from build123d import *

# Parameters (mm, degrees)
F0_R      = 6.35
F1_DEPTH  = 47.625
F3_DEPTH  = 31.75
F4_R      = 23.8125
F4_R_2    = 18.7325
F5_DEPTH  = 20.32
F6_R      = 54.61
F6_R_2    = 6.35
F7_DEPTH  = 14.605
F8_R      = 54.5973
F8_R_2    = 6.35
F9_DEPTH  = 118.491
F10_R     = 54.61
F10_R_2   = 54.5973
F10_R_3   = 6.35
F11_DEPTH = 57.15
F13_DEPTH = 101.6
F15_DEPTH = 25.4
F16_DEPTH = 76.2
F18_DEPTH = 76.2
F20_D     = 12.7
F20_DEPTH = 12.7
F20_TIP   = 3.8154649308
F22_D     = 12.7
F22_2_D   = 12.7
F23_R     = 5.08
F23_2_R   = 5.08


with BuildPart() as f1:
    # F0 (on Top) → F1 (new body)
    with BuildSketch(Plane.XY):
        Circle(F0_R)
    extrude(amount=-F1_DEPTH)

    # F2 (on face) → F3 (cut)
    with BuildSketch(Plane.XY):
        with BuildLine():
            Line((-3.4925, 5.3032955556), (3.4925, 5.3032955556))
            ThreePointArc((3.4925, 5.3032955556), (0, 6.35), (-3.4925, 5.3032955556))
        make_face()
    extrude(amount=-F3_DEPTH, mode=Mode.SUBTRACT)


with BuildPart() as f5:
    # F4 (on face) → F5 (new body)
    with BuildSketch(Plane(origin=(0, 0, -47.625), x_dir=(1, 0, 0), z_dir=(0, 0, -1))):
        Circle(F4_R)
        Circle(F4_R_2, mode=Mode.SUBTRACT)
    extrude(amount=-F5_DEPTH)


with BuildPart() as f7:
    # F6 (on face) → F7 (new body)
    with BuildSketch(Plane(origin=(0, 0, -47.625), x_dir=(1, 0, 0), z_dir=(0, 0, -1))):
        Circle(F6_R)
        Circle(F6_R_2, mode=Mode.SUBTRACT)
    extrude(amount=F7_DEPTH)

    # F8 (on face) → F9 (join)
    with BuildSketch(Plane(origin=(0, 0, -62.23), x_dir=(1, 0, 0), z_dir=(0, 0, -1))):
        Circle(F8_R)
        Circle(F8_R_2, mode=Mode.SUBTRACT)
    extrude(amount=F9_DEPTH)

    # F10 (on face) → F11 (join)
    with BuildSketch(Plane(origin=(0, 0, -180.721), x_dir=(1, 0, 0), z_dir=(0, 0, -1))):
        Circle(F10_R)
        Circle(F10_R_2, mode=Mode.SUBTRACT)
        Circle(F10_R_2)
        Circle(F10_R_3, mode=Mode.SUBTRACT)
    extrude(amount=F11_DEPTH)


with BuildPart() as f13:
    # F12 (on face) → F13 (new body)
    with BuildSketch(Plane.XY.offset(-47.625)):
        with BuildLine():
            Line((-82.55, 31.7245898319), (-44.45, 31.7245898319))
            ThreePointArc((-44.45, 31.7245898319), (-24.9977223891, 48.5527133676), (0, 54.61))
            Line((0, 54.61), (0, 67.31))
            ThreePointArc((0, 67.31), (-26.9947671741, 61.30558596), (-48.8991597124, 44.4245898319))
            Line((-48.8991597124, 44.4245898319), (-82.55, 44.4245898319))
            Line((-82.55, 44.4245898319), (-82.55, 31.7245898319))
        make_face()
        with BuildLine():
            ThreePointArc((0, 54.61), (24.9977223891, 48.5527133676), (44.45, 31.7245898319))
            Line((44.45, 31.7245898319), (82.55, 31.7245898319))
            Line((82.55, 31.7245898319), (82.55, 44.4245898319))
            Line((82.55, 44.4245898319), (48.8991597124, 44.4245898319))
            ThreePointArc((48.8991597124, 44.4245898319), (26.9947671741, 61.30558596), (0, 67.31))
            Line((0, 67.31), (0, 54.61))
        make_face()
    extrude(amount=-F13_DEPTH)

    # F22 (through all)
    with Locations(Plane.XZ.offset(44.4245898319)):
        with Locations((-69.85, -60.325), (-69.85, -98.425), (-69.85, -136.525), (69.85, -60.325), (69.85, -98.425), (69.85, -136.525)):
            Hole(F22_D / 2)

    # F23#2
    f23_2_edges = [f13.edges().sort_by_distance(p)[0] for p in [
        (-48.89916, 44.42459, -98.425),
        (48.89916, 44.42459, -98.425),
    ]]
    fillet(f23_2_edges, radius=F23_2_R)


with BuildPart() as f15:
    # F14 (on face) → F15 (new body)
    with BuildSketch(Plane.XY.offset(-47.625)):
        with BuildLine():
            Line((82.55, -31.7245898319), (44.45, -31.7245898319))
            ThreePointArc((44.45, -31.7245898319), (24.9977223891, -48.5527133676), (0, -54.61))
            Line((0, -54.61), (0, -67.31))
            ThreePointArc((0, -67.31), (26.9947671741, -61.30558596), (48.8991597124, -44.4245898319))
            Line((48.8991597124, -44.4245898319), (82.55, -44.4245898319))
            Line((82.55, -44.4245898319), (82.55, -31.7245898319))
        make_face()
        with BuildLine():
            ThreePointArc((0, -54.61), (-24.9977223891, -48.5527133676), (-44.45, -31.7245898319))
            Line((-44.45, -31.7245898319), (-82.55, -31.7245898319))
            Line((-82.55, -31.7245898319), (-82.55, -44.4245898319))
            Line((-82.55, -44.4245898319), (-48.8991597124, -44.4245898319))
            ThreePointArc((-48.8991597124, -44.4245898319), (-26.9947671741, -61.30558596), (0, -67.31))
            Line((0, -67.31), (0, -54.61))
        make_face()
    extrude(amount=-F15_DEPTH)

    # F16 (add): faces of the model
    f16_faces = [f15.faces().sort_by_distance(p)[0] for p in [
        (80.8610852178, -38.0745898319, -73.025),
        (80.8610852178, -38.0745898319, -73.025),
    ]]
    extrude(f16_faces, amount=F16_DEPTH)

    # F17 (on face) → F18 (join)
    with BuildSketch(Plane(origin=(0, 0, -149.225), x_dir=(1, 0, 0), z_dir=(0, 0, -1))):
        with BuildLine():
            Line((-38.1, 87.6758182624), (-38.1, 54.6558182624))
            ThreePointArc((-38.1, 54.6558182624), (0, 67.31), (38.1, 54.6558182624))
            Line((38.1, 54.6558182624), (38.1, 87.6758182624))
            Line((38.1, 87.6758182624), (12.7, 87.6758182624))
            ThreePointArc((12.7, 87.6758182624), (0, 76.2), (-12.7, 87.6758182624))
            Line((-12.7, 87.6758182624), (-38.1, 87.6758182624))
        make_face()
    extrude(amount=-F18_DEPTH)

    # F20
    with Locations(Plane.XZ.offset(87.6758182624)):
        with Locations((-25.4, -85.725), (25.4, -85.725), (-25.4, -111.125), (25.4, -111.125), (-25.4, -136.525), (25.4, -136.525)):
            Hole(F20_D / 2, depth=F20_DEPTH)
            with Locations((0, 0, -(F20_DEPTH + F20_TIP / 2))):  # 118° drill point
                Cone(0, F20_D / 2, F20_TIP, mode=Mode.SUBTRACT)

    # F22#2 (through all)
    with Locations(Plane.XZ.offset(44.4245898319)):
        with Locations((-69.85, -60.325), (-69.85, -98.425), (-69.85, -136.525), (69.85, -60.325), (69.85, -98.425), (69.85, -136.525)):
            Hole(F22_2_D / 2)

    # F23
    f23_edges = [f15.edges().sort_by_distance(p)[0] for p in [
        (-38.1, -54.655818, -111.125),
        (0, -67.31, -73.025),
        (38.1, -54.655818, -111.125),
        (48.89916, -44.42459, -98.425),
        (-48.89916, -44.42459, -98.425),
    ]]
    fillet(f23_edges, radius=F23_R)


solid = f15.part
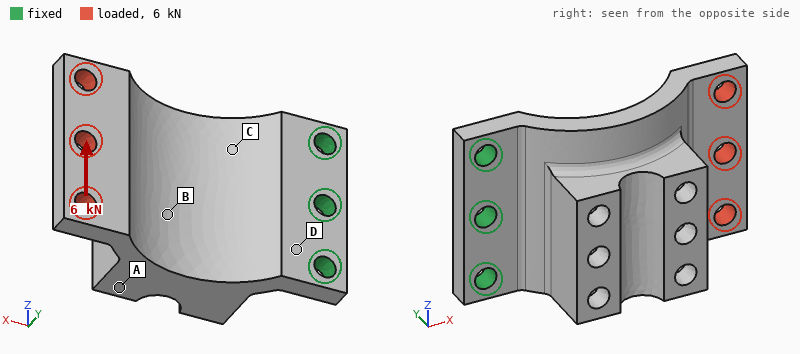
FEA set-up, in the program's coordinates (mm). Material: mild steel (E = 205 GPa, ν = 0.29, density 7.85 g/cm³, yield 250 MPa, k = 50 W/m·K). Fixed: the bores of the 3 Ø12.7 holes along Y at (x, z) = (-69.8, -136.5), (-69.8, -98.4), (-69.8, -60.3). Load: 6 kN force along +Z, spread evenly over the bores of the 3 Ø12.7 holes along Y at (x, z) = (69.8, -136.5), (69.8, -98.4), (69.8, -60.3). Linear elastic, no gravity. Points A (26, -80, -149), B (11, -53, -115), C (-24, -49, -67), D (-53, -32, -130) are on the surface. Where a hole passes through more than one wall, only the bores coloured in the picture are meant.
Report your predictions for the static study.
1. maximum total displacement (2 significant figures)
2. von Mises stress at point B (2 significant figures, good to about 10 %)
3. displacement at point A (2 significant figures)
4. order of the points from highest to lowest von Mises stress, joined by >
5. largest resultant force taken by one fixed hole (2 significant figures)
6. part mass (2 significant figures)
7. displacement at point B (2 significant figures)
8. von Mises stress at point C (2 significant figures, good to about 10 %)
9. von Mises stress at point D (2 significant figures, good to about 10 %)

0.14 mm
22 MPa
0.073 mm
C > D > B > A
11 kN
2.6 kg
0.042 mm
77 MPa
47 MPa
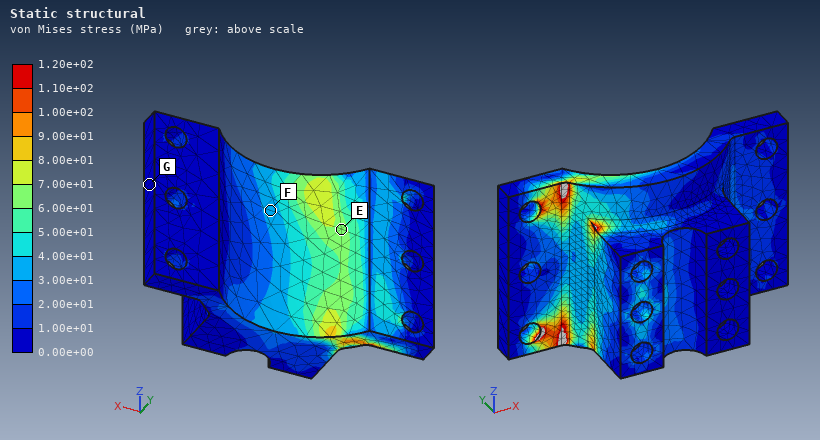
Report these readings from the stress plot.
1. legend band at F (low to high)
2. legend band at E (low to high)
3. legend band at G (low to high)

3.00e+01 to 4.00e+01 MPa
6.00e+01 to 7.00e+01 MPa
0.00e+00 to 1.00e+01 MPa
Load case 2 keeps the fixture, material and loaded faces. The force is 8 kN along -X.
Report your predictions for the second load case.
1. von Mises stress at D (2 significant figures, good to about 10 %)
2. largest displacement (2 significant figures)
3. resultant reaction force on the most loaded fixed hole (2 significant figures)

8.4 MPa
0.14 mm
2.8 kN
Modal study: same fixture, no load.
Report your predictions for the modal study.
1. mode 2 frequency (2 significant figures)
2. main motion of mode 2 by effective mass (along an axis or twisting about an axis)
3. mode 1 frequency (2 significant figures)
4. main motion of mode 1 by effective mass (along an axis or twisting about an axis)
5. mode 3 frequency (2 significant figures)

1400 Hz
along Z
410 Hz
along Y
2400 Hz
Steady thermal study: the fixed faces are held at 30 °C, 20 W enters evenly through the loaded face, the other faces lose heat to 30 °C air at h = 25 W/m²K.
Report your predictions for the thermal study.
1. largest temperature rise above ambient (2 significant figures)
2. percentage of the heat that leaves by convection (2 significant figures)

26 K
62 %
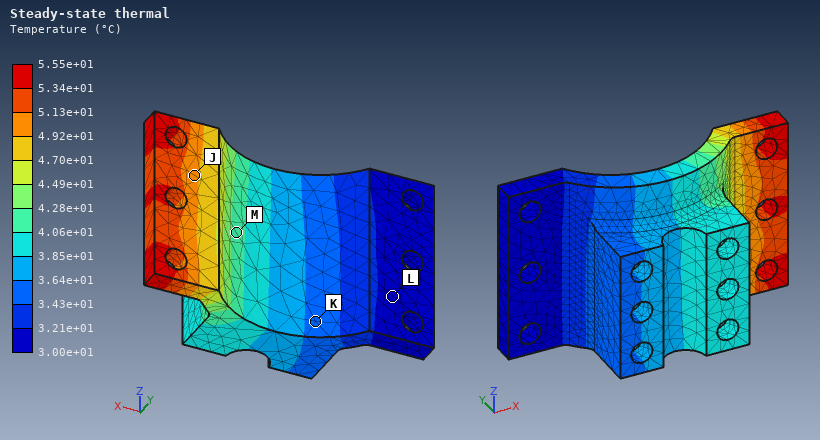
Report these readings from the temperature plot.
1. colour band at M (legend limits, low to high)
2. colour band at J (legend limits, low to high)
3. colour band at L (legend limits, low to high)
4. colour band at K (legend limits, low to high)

4.06e+01 to 4.28e+01 °C
4.92e+01 to 5.13e+01 °C
3.00e+01 to 3.21e+01 °C
3.43e+01 to 3.64e+01 °C
